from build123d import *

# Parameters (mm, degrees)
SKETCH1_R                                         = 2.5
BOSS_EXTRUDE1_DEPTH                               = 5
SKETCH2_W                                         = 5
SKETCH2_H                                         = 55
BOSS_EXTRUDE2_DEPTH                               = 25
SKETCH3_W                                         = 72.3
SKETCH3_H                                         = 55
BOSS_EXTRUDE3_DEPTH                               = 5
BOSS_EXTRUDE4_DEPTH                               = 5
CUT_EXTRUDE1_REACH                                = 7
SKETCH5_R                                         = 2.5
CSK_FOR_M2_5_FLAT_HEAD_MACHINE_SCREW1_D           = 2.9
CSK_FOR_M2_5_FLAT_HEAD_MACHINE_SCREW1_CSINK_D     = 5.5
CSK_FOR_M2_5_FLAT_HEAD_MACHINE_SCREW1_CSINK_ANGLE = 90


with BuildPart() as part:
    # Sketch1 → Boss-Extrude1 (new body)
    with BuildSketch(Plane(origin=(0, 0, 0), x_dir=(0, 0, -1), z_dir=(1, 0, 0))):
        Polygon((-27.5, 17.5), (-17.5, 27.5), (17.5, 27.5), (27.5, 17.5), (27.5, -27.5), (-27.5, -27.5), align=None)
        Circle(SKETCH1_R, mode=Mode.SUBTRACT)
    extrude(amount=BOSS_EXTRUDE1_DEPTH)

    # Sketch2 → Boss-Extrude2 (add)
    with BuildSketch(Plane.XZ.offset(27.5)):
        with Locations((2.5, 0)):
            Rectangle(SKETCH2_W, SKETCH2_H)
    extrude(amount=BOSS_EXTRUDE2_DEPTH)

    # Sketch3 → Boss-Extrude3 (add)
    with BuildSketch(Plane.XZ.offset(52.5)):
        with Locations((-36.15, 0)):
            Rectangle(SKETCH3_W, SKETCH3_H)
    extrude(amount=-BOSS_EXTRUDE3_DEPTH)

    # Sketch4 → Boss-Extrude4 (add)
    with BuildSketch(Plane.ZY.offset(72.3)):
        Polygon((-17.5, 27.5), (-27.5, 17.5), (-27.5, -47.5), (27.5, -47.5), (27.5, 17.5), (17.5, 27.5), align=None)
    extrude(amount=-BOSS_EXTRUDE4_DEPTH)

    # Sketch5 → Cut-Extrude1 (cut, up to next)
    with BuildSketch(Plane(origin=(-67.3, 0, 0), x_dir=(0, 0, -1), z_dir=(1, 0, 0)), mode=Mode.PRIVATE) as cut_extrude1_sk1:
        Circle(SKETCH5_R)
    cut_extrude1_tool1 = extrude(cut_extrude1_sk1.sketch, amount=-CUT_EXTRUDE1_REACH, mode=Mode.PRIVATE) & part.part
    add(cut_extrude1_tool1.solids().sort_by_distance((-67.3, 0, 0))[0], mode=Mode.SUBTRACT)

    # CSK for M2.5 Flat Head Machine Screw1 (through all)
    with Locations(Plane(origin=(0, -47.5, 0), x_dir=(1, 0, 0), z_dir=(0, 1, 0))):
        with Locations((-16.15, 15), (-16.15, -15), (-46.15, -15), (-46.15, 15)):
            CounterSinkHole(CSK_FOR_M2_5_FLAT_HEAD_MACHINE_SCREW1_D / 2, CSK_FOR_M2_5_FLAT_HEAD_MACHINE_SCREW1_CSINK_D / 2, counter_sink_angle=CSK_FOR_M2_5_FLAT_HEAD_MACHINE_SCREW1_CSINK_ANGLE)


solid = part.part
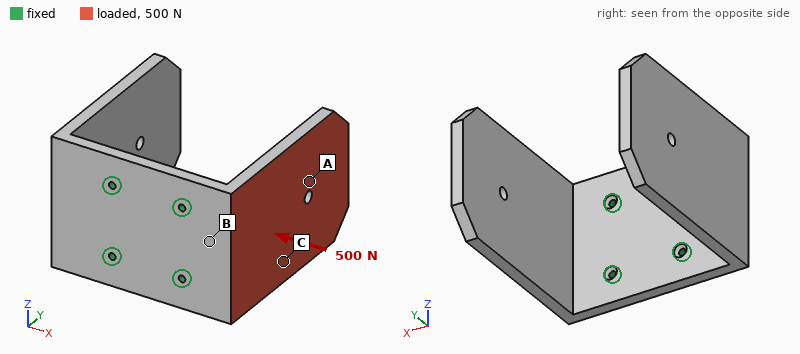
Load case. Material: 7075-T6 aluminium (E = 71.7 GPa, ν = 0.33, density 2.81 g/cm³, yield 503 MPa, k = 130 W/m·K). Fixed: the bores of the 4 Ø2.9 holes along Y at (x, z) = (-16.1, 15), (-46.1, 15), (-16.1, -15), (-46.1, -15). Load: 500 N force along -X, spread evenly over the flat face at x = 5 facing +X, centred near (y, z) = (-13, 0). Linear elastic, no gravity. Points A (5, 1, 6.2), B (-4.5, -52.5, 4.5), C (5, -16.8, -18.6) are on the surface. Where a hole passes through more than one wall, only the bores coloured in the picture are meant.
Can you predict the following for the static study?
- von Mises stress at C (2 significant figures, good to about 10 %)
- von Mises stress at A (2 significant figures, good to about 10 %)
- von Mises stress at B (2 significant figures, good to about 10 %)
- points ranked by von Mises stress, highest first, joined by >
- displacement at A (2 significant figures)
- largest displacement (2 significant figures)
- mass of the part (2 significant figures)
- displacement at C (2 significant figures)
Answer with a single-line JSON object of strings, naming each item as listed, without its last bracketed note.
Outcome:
{"von Mises stress at C": "25 MPa", "von Mises stress at A": "9.9 MPa", "von Mises stress at B": "69 MPa", "points ranked by von Mises stress, highest first, joined by >": "B > C > A", "displacement at A": "0.79 mm", "largest displacement": "1.3 mm", "mass of the part": "170 g", "displacement at C": "0.47 mm"}
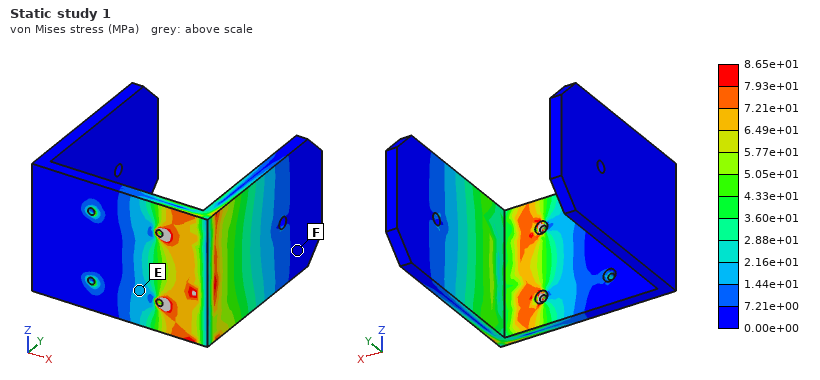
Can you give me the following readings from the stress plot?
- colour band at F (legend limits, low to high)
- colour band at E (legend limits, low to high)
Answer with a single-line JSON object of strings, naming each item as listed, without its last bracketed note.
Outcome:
{"colour band at F": "0.00e+00 to 7.21e+00 MPa", "colour band at E": "1.44e+01 to 2.16e+01 MPa"}
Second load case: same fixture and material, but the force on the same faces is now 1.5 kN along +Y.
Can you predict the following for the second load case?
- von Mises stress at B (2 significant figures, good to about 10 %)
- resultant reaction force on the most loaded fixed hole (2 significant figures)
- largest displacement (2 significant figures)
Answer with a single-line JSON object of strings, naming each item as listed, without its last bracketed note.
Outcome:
{"von Mises stress at B": "57 MPa", "resultant reaction force on the most loaded fixed hole": "1.1 kN", "largest displacement": "0.97 mm"}
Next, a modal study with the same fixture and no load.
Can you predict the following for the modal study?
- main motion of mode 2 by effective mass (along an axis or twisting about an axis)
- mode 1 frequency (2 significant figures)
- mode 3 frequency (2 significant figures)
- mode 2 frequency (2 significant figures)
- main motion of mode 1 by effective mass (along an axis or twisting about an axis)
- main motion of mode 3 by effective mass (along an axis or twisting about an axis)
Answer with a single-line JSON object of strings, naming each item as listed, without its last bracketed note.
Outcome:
{"main motion of mode 2 by effective mass": "along X", "mode 1 frequency": "470 Hz", "mode 3 frequency": "1000 Hz", "mode 2 frequency": "500 Hz", "main motion of mode 1 by effective mass": "along X", "main motion of mode 3 by effective mass": "along Z"}
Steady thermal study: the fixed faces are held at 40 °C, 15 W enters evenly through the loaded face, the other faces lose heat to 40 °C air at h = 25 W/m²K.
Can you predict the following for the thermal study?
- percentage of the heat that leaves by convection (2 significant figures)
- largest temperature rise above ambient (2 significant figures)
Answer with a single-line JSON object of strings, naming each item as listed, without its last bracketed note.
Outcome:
{"percentage of the heat that leaves by convection": "17 %", "largest temperature rise above ambient": "20 K"}
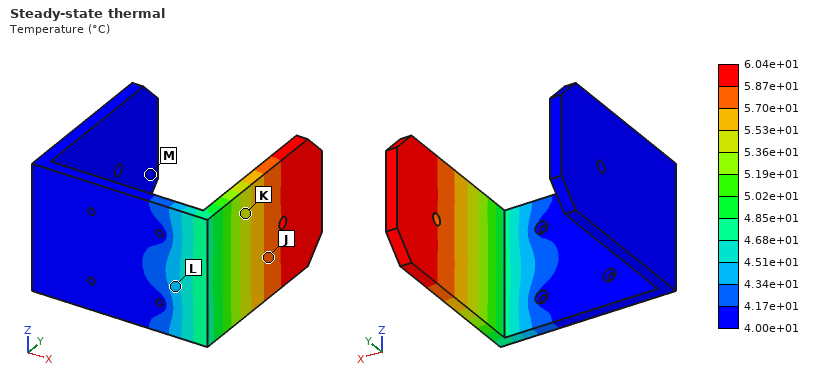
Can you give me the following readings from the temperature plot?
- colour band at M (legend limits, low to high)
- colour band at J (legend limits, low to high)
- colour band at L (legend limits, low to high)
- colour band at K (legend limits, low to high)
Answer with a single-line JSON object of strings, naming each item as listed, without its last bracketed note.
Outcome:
{"colour band at M": "4.00e+01 to 4.17e+01 °C", "colour band at J": "5.70e+01 to 5.87e+01 °C", "colour band at L": "4.34e+01 to 4.51e+01 °C", "colour band at K": "5.36e+01 to 5.53e+01 °C"}
